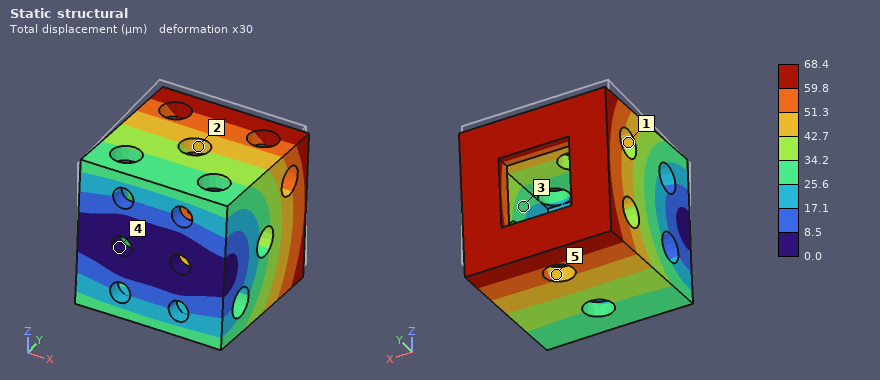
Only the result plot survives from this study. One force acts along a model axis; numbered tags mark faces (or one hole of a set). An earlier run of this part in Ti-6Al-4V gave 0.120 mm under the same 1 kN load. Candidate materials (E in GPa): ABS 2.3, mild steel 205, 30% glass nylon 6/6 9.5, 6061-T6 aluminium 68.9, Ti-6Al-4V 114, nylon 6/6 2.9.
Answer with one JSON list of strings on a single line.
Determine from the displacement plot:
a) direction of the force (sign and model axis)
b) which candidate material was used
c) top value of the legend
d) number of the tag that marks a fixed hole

["-Z", "mild steel", "68.4 µm", "4"]
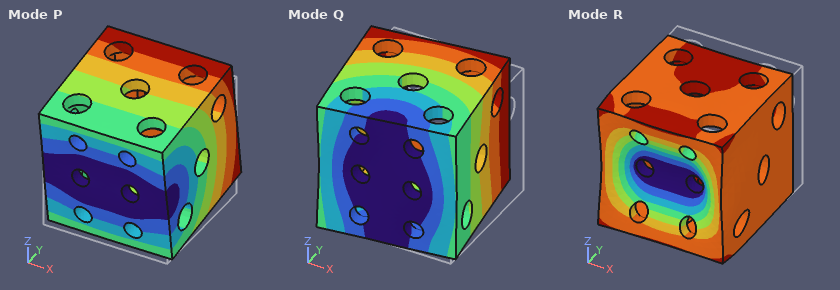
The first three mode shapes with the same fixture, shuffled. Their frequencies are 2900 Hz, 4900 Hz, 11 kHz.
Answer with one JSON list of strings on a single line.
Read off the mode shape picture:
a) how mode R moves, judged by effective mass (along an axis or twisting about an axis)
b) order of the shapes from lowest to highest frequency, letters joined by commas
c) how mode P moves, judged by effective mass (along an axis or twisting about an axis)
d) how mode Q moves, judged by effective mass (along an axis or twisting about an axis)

["along Y", "P, Q, R", "along Z", "along X"]
